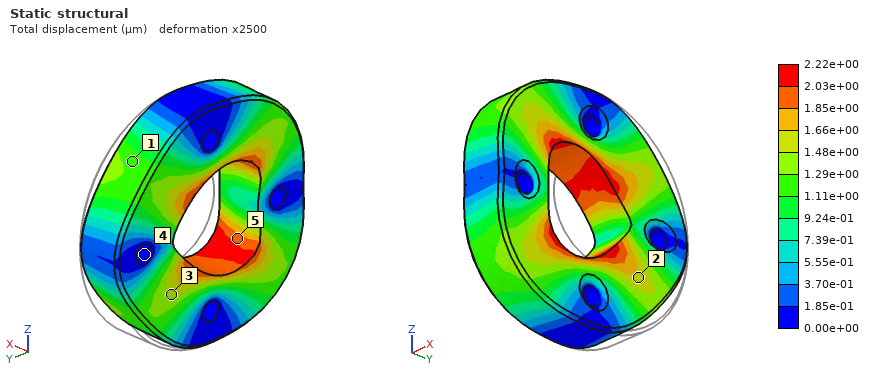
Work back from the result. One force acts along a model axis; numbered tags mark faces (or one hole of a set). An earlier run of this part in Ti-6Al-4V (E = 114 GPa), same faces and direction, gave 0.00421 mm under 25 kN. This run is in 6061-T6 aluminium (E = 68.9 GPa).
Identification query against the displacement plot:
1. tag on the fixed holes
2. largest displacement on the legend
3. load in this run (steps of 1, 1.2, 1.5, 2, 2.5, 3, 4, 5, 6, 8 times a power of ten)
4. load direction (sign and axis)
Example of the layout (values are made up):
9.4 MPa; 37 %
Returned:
4; 2.22e+00 µm; 8 kN; -Y
